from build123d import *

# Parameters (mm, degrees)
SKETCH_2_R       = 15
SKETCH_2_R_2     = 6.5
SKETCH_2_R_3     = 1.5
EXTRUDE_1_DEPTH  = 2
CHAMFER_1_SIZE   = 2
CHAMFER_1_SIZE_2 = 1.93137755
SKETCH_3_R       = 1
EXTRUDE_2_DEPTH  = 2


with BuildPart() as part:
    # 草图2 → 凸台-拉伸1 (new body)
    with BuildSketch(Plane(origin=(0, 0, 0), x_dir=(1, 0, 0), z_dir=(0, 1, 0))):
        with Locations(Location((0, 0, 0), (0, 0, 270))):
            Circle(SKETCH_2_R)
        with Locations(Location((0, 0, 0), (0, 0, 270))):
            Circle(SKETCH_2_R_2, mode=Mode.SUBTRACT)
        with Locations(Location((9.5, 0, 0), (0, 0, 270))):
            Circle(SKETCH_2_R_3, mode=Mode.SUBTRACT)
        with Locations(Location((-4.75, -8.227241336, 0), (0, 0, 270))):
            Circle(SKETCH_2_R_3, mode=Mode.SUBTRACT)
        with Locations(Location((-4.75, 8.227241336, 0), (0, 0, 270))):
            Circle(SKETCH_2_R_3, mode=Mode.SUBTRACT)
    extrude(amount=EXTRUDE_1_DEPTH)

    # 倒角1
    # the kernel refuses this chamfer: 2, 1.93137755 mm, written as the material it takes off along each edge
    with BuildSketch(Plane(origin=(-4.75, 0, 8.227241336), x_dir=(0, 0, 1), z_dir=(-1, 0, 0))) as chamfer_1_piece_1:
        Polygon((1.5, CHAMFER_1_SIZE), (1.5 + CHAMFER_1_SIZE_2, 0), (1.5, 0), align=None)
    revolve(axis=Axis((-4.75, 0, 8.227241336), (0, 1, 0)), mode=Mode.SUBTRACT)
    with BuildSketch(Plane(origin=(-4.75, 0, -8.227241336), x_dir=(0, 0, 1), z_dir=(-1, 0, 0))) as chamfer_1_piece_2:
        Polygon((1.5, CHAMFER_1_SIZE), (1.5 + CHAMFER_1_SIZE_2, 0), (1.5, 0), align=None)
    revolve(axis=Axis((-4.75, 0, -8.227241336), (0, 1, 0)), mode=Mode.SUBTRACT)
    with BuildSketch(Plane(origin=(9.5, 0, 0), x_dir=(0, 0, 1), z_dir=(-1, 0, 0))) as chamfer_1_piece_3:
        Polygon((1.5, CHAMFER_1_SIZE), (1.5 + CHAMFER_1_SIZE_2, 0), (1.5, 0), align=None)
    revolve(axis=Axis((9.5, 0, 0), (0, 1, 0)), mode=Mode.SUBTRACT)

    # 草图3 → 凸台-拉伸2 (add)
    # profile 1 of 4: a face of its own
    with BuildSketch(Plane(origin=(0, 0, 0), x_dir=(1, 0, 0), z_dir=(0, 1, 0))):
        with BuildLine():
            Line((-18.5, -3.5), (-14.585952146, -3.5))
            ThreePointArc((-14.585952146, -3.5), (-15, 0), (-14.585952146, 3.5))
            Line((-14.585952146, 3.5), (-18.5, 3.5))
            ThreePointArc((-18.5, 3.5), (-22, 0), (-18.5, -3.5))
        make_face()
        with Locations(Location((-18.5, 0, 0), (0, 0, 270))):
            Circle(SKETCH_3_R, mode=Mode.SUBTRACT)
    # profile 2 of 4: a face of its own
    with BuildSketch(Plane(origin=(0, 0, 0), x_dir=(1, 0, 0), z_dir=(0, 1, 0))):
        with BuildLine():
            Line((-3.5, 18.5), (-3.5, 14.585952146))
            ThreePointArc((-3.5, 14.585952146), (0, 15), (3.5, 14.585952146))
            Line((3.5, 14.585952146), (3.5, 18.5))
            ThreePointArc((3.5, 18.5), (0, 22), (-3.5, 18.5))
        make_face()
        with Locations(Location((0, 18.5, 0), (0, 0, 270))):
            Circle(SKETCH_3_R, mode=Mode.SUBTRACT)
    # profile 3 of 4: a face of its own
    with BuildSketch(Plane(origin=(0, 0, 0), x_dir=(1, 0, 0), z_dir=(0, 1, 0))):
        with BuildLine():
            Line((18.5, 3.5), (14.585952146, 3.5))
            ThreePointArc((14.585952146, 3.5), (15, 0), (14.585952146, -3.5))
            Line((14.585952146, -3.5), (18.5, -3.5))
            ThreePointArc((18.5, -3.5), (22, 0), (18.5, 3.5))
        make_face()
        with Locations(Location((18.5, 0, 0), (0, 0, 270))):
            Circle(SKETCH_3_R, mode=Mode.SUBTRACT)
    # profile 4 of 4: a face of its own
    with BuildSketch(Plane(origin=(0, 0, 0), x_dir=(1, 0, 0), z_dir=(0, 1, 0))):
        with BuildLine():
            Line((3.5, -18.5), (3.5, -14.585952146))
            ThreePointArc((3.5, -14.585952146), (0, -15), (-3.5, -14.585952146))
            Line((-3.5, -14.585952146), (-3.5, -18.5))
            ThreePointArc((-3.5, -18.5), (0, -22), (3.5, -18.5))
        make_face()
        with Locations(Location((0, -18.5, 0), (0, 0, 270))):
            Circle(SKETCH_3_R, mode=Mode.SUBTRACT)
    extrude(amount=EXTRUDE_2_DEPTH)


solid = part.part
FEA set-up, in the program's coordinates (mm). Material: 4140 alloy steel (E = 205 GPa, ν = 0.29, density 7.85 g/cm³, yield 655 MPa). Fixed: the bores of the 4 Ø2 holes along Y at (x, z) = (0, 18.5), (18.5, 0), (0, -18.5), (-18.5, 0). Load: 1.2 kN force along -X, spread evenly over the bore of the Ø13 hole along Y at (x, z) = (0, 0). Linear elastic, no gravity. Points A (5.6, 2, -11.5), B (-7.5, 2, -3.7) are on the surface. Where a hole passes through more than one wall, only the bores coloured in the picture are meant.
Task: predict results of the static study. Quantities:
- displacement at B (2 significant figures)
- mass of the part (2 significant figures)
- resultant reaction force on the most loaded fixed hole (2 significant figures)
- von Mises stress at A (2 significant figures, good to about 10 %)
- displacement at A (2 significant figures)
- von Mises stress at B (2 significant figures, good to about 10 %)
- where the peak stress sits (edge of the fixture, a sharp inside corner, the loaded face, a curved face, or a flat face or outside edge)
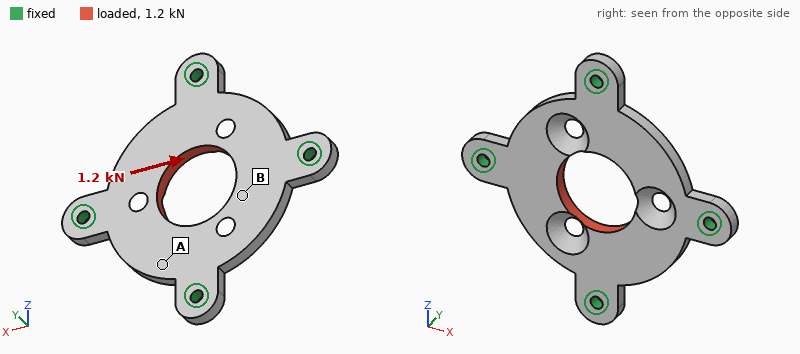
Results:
2.2 µm
11 g
470 N
12 MPa
2.1 µm
30 MPa
a curved face
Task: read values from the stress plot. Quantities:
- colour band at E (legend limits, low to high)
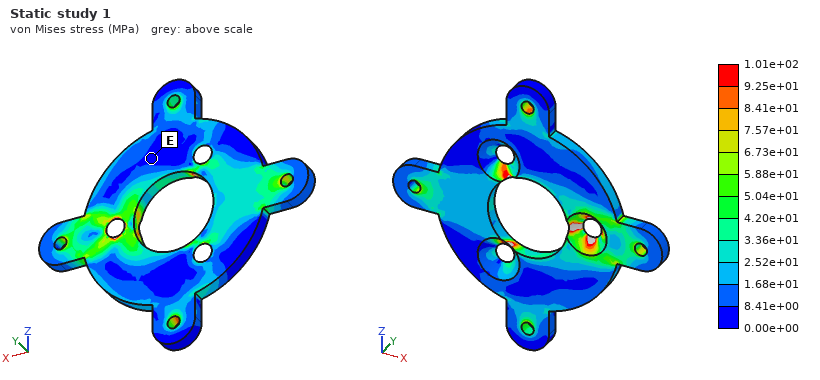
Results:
0.00e+00 to 8.41e+00 MPa
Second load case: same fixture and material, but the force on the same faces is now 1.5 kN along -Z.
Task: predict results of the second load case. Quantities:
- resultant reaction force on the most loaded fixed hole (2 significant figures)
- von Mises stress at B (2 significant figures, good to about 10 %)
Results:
550 N
33 MPa
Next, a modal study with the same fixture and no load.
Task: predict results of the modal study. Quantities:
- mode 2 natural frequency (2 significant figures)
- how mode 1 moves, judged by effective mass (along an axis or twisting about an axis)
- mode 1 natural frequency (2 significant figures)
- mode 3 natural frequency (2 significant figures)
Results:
15 kHz
along Y
11 kHz
16 kHz
